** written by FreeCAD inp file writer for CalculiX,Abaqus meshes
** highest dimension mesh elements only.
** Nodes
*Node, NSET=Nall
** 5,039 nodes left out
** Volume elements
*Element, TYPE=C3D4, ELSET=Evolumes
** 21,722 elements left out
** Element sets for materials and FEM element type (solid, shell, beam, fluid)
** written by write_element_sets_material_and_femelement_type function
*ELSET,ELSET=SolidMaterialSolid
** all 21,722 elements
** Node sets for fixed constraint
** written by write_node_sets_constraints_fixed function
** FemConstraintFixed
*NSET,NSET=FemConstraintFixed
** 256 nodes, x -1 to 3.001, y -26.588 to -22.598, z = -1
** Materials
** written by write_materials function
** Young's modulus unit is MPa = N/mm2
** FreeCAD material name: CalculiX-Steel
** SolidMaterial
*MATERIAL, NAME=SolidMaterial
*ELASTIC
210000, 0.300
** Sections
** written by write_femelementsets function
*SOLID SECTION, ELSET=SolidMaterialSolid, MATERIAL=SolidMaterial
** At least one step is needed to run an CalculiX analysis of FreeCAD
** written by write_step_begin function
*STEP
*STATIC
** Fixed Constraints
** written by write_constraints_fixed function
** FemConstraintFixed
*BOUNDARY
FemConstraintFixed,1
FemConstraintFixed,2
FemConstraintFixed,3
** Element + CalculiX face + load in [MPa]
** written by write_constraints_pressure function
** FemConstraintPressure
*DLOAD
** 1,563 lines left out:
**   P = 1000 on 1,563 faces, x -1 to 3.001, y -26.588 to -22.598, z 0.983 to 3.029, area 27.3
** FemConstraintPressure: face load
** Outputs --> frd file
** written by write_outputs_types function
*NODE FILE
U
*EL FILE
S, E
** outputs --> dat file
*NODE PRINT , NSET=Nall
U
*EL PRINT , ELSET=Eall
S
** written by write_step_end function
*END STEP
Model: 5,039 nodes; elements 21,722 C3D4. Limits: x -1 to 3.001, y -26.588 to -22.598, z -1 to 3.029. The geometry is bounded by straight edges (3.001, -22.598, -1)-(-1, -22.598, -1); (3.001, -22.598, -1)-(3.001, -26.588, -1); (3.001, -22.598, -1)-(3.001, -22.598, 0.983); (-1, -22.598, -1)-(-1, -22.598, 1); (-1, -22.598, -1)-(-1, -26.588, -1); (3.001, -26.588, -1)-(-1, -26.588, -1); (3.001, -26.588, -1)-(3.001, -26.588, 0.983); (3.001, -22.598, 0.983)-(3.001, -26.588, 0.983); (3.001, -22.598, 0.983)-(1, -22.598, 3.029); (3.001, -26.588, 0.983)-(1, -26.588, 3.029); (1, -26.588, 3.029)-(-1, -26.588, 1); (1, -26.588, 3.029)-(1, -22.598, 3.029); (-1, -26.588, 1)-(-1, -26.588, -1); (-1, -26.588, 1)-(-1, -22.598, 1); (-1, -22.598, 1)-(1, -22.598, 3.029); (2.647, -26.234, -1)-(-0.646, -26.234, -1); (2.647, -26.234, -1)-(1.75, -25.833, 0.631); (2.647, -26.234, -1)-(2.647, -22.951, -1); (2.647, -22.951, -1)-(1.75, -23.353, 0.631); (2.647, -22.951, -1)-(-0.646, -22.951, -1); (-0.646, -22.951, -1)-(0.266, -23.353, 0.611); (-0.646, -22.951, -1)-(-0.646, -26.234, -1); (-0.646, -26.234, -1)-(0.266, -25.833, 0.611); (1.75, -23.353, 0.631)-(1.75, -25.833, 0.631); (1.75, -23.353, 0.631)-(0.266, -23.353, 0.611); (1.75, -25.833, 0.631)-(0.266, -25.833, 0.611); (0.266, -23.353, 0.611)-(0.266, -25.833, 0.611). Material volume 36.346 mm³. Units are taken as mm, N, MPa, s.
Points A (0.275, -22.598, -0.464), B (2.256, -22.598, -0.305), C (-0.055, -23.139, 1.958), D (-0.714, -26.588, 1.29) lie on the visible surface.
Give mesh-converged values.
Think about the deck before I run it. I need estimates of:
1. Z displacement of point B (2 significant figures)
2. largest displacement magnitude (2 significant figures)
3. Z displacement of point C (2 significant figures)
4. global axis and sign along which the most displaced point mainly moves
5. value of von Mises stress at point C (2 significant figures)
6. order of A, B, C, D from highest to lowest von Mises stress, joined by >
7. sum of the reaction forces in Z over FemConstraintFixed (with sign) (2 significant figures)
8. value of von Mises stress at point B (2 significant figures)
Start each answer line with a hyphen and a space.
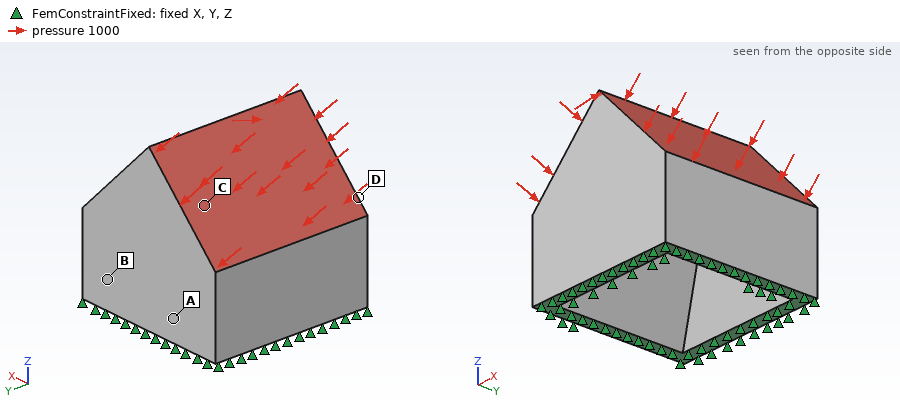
- -0.0071 mm
- 0.028 mm
- -0.022 mm
- -Z
- 1200 MPa
- A > B > C > D
- 16000 N
- 1700 MPa
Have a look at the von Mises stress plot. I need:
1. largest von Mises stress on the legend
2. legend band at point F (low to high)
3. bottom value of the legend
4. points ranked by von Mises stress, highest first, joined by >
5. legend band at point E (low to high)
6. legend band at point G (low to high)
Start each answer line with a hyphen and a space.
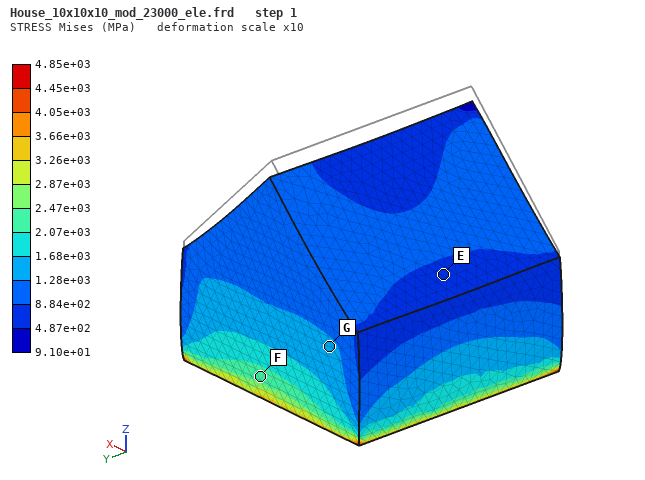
- 4.85e+03 MPa
- 2.07e+03 to 2.47e+03 MPa
- 9.10e+01 MPa
- F > G > E
- 4.87e+02 to 8.84e+02 MPa
- 1.28e+03 to 1.68e+03 MPa
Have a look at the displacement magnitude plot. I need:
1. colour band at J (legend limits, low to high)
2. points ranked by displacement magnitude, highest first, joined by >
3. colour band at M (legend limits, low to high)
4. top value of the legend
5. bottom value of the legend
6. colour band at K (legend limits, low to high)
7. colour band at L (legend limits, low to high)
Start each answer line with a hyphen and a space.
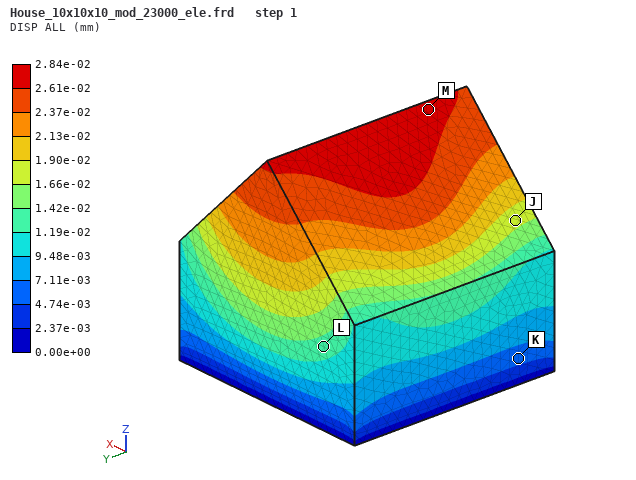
- 1.66e-02 to 1.90e-02 mm
- M > J > L > K
- 2.61e-02 to 2.84e-02 mm
- 2.84e-02 mm
- 0.00e+00 mm
- 4.74e-03 to 7.11e-03 mm
- 1.19e-02 to 1.42e-02 mm
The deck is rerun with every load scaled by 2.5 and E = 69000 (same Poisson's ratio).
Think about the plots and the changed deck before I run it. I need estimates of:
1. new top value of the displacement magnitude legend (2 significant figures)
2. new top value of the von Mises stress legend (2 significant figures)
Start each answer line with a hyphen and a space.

- 0.22 mm
- 12000 MPa
